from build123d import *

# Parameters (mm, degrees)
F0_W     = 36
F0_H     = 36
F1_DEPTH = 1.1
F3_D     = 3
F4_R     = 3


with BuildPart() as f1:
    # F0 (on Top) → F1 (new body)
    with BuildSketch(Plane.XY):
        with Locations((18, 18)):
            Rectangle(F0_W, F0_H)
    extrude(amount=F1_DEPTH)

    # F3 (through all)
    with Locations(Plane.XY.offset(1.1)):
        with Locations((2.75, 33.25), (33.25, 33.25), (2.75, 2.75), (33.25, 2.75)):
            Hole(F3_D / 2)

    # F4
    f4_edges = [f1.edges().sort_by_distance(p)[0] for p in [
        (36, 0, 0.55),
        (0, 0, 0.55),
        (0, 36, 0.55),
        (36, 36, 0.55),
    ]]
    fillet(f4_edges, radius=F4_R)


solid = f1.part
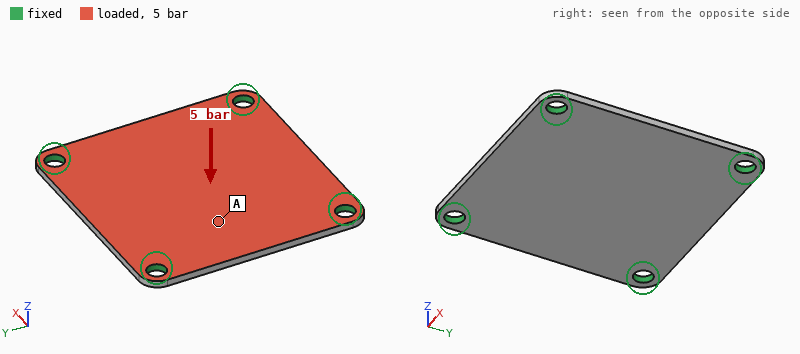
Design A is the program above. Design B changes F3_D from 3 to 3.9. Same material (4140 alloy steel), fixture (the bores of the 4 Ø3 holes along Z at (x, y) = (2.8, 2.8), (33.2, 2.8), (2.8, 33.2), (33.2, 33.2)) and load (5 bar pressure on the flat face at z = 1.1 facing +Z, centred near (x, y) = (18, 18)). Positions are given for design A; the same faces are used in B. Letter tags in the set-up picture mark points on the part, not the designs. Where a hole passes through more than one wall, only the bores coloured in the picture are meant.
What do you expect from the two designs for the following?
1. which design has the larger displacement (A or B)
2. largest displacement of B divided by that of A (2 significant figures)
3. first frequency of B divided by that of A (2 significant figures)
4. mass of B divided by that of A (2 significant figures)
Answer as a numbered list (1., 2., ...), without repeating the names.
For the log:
1. A
2. 0.88
3. 1.1
4. 0.98
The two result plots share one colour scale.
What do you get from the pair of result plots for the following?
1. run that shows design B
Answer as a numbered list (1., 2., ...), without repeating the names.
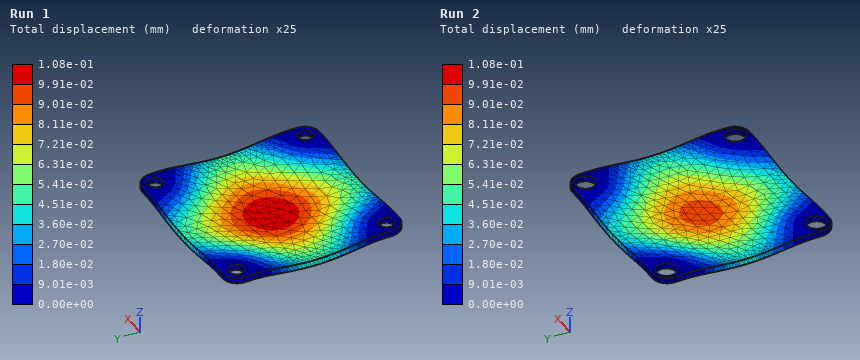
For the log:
1. Run 2
